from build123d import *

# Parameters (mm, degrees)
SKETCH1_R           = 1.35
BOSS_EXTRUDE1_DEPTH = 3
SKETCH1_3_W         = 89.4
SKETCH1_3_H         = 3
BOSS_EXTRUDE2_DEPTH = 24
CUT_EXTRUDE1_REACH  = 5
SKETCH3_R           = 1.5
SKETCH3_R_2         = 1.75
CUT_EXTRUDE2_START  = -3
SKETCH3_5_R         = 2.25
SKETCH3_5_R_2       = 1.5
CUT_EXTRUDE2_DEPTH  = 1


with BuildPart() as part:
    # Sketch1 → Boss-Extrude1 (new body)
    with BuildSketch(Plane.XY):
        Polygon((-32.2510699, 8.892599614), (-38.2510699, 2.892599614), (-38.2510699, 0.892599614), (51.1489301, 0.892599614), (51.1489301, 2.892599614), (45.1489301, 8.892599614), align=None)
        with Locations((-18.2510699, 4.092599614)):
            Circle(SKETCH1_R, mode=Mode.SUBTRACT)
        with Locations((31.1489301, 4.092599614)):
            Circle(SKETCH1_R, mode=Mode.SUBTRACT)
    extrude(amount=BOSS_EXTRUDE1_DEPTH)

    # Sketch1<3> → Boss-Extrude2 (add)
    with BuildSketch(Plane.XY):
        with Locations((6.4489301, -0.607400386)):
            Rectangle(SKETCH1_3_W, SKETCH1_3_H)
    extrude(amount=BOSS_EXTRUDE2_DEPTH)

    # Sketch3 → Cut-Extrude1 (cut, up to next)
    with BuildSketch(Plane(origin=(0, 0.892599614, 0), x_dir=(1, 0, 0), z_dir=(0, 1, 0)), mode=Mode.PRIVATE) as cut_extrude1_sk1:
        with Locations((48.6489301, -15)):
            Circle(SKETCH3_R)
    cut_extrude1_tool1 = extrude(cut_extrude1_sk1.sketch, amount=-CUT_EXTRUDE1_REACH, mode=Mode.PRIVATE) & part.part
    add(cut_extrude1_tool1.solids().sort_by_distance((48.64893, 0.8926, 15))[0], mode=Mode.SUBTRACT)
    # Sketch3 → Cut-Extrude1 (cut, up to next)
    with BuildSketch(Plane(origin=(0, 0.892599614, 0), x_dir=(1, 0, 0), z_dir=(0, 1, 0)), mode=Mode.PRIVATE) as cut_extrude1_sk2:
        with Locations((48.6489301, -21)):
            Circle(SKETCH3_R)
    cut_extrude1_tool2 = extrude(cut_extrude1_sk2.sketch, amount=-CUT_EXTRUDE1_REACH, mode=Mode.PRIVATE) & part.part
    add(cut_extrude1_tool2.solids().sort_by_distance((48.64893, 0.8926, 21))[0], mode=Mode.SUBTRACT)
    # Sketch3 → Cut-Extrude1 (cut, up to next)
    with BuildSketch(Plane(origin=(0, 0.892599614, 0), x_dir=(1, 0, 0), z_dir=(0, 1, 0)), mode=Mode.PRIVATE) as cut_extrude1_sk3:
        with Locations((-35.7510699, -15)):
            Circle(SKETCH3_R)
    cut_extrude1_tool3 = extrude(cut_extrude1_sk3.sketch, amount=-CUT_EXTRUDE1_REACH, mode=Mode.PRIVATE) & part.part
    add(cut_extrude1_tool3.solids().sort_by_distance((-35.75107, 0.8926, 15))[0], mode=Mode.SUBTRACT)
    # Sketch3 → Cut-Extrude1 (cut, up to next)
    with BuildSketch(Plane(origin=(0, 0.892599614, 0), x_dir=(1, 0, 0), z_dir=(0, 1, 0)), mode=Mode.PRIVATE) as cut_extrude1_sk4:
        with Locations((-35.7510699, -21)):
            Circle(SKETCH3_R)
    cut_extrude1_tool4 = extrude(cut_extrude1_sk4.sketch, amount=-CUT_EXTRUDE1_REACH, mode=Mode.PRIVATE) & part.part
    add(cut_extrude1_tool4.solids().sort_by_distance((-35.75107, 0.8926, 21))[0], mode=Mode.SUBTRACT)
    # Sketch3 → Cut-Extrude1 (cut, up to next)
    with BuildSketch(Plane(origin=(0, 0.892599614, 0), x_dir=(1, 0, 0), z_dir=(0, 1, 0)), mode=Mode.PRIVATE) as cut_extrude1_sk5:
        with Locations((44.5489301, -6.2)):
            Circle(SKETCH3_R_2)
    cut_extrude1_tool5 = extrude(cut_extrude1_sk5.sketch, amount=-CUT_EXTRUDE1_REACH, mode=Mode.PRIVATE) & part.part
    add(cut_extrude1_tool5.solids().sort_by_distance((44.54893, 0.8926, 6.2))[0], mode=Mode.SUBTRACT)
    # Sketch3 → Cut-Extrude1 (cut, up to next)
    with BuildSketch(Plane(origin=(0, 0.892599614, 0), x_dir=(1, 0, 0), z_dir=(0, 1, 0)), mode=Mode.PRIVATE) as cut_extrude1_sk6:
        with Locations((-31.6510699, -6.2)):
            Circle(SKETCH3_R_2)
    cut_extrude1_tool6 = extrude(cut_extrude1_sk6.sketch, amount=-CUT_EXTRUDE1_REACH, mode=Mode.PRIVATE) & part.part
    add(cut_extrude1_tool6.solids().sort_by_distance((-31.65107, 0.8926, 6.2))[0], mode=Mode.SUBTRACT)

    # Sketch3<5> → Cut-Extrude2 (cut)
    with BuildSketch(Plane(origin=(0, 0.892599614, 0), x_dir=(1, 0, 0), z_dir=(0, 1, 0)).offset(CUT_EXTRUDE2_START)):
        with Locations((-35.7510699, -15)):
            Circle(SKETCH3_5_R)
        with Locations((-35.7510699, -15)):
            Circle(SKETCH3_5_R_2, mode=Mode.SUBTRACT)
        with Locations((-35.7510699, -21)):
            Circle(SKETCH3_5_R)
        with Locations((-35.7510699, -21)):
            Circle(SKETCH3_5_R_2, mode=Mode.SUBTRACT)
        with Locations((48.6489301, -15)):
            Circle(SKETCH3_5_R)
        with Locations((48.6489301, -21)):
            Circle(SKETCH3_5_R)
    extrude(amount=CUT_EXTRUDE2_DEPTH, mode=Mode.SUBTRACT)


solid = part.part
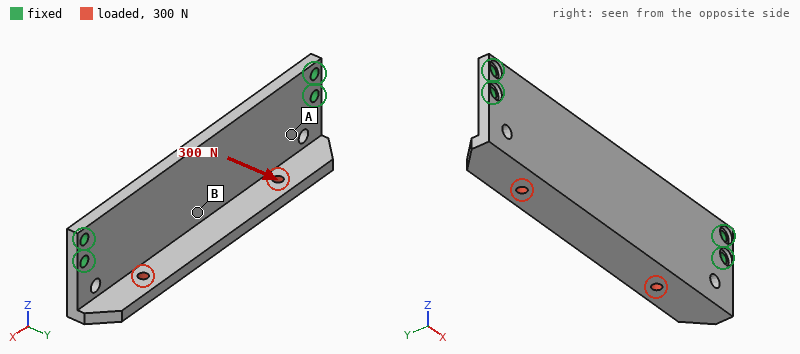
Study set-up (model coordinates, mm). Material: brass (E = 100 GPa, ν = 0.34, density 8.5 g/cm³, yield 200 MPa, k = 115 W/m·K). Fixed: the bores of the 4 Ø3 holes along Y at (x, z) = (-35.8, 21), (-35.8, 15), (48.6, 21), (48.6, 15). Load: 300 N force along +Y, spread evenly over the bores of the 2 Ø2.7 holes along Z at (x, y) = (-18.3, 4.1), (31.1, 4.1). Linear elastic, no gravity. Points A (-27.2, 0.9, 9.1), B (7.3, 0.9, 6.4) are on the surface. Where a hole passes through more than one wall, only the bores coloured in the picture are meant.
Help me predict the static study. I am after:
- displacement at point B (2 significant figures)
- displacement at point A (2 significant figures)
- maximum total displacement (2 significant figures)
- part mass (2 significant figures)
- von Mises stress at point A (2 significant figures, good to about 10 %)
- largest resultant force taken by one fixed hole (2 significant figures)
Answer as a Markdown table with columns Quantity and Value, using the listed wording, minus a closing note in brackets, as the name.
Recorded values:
| Quantity | Value |
|---|---|
| displacement at point B | 62 µm |
| displacement at point A | 28 µm |
| maximum total displacement | 97 µm |
| part mass | 70 g |
| von Mises stress at point A | 29 MPa |
| largest resultant force taken by one fixed hole | 300 N |
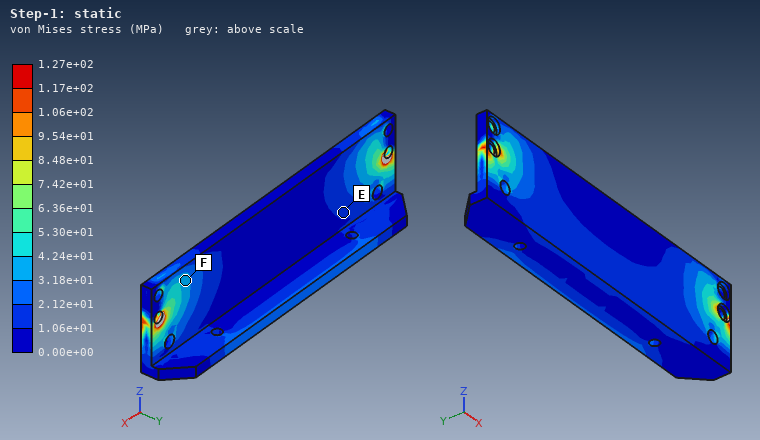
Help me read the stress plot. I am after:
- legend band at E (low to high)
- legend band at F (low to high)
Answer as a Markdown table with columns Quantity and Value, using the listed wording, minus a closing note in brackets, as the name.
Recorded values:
| Quantity | Value |
|---|---|
| legend band at E | 1.06e+01 to 2.12e+01 MPa |
| legend band at F | 3.18e+01 to 4.24e+01 MPa |
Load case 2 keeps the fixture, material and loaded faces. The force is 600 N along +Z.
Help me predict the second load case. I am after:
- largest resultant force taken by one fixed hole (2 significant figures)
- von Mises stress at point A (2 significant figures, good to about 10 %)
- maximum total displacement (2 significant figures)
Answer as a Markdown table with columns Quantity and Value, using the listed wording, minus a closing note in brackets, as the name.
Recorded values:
| Quantity | Value |
|---|---|
| largest resultant force taken by one fixed hole | 270 N |
| von Mises stress at point A | 39 MPa |
| maximum total displacement | 75 µm |
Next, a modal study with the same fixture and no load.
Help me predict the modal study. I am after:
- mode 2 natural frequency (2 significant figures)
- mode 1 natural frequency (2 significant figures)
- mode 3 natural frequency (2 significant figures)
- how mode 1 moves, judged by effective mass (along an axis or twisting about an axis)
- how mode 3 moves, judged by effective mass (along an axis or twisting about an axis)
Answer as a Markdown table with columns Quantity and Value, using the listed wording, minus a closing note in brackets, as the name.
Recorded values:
| Quantity | Value |
|---|---|
| mode 2 natural frequency | 2300 Hz |
| mode 1 natural frequency | 1600 Hz |
| mode 3 natural frequency | 3700 Hz |
| how mode 1 moves, judged by effective mass | along Y |
| how mode 3 moves, judged by effective mass | twisting about Z |
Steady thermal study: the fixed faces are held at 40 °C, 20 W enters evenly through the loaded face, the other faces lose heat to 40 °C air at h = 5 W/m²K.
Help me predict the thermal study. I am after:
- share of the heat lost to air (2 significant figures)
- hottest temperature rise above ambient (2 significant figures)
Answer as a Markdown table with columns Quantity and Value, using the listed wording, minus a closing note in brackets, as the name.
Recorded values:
| Quantity | Value |
|---|---|
| share of the heat lost to air | 3.5 % |
| hottest temperature rise above ambient | 39 K |
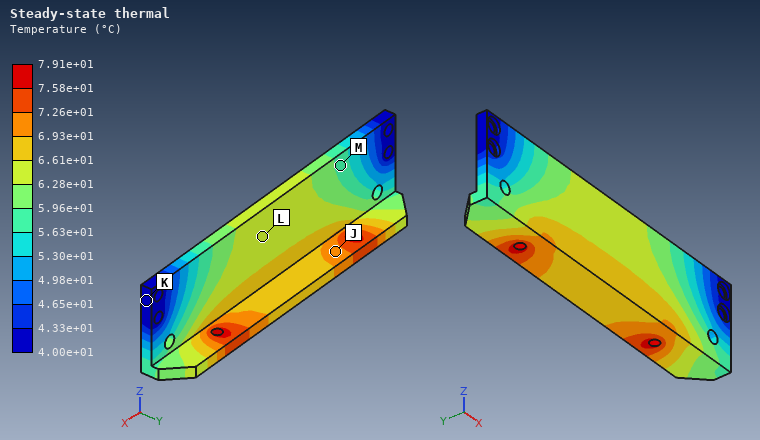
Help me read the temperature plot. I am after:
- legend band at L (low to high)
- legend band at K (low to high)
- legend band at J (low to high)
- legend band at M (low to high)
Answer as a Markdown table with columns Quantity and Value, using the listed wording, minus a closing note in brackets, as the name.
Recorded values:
| Quantity | Value |
|---|---|
| legend band at L | 6.28e+01 to 6.61e+01 °C |
| legend band at K | 4.00e+01 to 4.33e+01 °C |
| legend band at J | 6.93e+01 to 7.26e+01 °C |
| legend band at M | 5.63e+01 to 5.96e+01 °C |
